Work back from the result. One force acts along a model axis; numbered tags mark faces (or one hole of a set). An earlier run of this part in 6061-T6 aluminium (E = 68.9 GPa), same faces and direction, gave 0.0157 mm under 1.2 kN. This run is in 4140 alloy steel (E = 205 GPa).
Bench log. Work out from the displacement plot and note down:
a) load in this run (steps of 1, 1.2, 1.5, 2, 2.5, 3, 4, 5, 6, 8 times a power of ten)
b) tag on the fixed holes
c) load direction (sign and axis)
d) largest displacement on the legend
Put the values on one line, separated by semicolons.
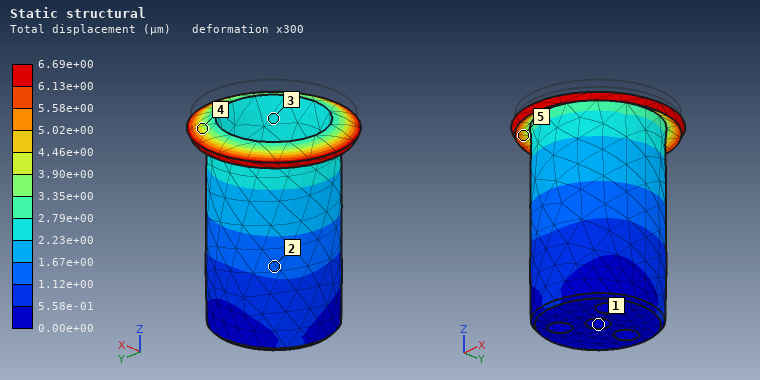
1.5 kN; 1; -Z; 6.69e+00 µm
